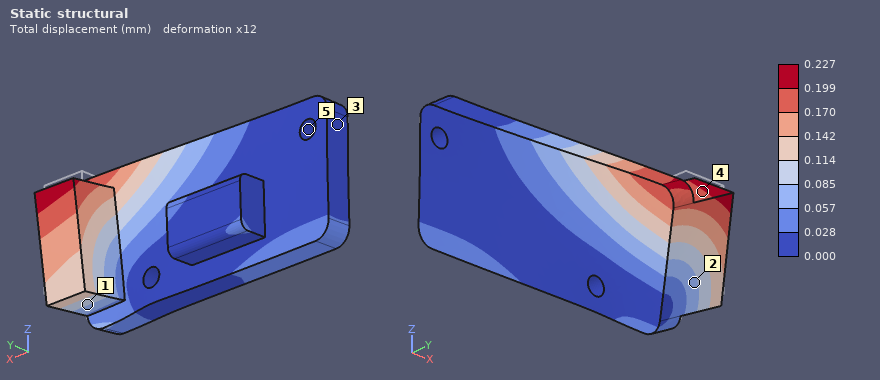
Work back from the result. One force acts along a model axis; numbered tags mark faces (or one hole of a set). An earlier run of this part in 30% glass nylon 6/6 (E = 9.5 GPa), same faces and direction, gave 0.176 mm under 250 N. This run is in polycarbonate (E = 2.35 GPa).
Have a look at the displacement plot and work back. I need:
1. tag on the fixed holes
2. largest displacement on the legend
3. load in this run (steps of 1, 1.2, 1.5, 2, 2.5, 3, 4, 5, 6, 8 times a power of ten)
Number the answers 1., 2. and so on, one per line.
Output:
1. 5
2. 0.227 mm
3. 80 N
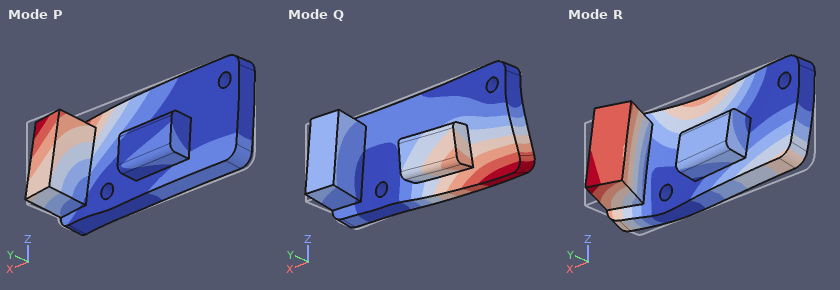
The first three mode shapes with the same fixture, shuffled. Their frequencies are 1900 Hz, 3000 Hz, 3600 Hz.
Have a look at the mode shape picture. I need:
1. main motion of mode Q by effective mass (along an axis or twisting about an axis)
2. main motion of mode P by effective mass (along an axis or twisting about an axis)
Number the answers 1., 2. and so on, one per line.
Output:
1. along Y
2. along Y
